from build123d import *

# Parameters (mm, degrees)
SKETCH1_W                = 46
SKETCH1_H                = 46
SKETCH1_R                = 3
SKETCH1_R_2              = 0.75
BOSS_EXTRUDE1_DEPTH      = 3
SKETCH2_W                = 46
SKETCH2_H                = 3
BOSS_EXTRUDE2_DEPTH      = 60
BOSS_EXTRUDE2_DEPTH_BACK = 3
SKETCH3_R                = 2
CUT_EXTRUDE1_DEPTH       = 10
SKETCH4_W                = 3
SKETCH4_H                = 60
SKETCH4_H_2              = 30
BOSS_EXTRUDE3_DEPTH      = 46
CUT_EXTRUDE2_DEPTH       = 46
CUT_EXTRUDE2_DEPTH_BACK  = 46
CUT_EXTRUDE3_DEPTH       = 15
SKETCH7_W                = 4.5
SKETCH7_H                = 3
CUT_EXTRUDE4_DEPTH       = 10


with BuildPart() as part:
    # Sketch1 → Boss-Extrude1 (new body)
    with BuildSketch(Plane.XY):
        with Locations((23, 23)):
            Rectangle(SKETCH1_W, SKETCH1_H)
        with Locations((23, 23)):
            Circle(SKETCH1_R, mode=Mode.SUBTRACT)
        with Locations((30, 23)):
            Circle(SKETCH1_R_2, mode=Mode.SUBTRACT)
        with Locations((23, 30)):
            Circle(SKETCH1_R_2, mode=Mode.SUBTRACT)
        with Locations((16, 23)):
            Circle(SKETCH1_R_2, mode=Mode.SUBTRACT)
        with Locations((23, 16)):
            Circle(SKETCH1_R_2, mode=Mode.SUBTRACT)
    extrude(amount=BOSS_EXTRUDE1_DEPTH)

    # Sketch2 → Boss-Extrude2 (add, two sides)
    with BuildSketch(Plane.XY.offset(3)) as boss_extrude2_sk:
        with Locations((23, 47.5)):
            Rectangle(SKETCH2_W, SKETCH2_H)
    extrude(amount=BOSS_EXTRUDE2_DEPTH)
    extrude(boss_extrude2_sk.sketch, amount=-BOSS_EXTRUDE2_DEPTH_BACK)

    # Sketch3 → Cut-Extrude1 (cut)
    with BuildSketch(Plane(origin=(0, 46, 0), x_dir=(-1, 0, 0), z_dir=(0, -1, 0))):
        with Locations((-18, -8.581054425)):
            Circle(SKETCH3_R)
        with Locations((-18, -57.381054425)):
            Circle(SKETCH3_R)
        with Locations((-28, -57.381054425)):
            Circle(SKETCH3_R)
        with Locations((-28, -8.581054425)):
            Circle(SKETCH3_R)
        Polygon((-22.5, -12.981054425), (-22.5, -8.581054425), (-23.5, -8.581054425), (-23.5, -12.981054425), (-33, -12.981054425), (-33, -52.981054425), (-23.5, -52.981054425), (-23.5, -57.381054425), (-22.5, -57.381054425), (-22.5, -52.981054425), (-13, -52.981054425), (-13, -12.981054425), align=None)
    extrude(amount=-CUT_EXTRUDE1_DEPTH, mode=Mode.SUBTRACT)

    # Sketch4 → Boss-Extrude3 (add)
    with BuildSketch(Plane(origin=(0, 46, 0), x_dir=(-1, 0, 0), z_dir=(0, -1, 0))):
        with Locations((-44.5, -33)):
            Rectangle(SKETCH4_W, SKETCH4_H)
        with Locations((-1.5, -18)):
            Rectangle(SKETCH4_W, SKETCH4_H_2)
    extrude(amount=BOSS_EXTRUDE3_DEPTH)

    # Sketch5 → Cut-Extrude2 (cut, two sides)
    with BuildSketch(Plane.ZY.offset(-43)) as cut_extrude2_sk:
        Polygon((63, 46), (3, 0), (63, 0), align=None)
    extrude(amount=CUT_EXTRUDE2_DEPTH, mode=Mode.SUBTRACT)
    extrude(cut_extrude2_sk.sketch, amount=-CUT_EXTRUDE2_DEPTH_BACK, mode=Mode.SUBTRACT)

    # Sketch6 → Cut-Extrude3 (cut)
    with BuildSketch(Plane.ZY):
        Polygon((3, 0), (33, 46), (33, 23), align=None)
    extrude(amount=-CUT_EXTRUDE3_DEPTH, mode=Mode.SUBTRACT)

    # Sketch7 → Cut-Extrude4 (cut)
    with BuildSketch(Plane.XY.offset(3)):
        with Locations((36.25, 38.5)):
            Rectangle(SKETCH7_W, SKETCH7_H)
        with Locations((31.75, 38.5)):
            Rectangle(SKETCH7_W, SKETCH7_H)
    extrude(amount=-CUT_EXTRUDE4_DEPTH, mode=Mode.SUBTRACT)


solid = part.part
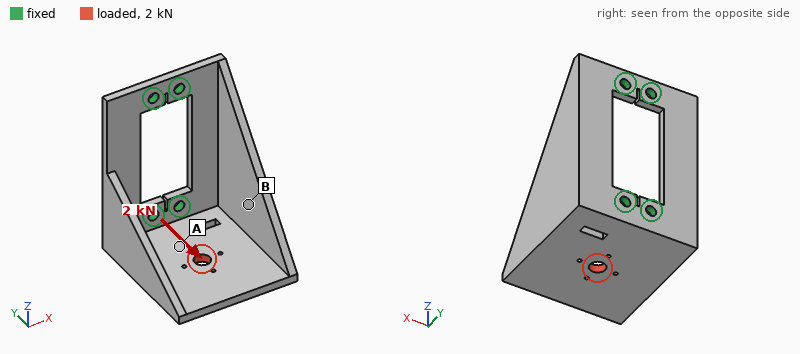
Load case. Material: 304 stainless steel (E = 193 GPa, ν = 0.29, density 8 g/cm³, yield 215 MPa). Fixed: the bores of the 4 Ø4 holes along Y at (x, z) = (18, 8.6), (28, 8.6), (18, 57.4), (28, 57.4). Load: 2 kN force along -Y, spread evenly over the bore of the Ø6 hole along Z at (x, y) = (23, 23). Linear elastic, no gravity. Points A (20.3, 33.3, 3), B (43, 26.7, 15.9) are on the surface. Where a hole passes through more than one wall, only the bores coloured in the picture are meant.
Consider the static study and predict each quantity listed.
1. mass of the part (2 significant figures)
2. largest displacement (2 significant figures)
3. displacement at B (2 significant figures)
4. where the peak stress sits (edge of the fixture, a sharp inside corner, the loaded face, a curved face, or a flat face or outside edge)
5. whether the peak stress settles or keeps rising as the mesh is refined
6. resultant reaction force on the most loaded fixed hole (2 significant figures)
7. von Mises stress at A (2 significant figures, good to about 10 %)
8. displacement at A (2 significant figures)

150 g
41 µm
12 µm
edge of the fixture
keeps rising
1.1 kN
40 MPa
19 µm
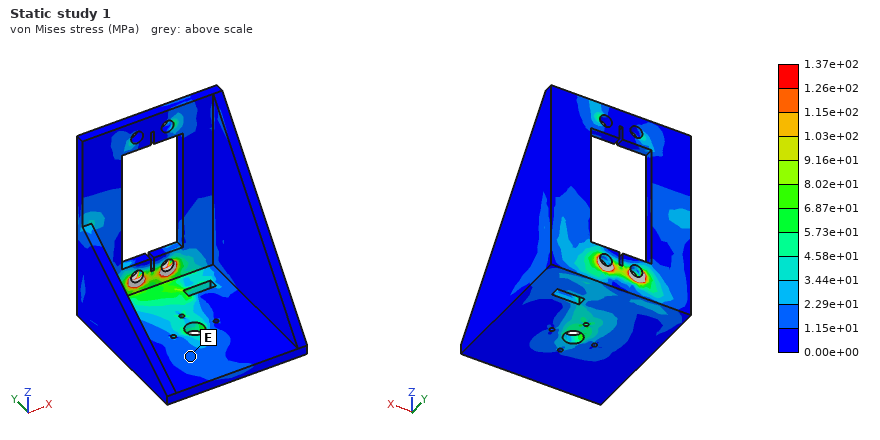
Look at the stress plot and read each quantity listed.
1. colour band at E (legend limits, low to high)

1.15e+01 to 2.29e+01 MPa
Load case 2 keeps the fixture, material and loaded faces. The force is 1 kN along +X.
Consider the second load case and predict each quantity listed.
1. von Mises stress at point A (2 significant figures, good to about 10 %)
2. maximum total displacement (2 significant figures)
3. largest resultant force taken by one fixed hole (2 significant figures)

33 MPa
0.12 mm
1.6 kN
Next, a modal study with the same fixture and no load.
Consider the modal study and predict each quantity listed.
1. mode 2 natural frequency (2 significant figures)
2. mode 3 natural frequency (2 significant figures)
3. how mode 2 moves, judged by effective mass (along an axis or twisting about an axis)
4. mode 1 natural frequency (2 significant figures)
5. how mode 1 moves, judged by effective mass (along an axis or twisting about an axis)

2000 Hz
3100 Hz
along Z
1700 Hz
along X
